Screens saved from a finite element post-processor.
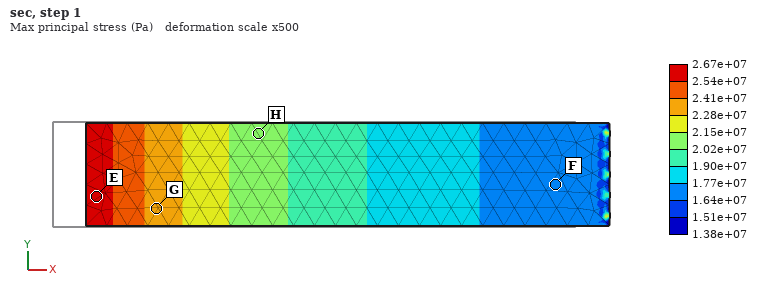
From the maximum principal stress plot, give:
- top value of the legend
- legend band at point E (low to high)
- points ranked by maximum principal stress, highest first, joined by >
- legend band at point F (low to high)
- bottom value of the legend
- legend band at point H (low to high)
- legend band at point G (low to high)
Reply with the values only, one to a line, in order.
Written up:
2.67e+07 Pa
2.54e+07 to 2.67e+07 Pa
E > G > H > F
1.64e+07 to 1.77e+07 Pa
1.38e+07 Pa
2.02e+07 to 2.15e+07 Pa
2.28e+07 to 2.41e+07 Pa
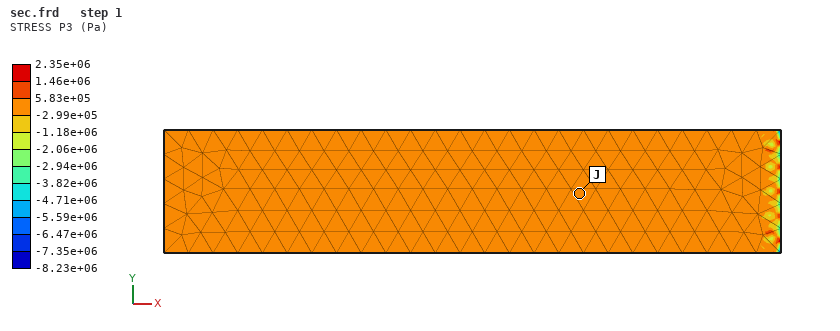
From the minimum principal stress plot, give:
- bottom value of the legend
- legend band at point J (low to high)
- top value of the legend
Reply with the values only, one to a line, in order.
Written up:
-8.23e+06 Pa
-2.99e+05 to 5.83e+05 Pa
2.35e+06 Pa
